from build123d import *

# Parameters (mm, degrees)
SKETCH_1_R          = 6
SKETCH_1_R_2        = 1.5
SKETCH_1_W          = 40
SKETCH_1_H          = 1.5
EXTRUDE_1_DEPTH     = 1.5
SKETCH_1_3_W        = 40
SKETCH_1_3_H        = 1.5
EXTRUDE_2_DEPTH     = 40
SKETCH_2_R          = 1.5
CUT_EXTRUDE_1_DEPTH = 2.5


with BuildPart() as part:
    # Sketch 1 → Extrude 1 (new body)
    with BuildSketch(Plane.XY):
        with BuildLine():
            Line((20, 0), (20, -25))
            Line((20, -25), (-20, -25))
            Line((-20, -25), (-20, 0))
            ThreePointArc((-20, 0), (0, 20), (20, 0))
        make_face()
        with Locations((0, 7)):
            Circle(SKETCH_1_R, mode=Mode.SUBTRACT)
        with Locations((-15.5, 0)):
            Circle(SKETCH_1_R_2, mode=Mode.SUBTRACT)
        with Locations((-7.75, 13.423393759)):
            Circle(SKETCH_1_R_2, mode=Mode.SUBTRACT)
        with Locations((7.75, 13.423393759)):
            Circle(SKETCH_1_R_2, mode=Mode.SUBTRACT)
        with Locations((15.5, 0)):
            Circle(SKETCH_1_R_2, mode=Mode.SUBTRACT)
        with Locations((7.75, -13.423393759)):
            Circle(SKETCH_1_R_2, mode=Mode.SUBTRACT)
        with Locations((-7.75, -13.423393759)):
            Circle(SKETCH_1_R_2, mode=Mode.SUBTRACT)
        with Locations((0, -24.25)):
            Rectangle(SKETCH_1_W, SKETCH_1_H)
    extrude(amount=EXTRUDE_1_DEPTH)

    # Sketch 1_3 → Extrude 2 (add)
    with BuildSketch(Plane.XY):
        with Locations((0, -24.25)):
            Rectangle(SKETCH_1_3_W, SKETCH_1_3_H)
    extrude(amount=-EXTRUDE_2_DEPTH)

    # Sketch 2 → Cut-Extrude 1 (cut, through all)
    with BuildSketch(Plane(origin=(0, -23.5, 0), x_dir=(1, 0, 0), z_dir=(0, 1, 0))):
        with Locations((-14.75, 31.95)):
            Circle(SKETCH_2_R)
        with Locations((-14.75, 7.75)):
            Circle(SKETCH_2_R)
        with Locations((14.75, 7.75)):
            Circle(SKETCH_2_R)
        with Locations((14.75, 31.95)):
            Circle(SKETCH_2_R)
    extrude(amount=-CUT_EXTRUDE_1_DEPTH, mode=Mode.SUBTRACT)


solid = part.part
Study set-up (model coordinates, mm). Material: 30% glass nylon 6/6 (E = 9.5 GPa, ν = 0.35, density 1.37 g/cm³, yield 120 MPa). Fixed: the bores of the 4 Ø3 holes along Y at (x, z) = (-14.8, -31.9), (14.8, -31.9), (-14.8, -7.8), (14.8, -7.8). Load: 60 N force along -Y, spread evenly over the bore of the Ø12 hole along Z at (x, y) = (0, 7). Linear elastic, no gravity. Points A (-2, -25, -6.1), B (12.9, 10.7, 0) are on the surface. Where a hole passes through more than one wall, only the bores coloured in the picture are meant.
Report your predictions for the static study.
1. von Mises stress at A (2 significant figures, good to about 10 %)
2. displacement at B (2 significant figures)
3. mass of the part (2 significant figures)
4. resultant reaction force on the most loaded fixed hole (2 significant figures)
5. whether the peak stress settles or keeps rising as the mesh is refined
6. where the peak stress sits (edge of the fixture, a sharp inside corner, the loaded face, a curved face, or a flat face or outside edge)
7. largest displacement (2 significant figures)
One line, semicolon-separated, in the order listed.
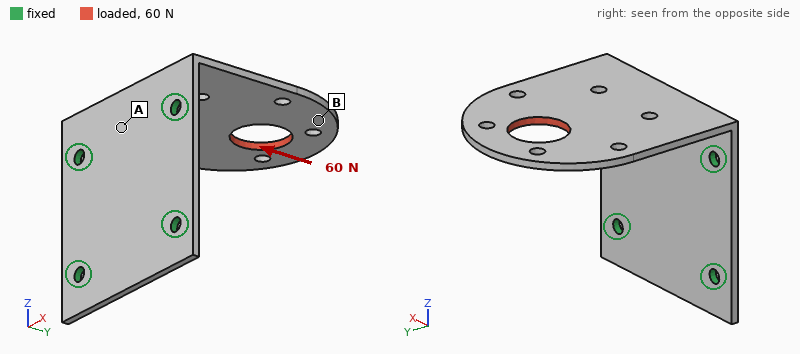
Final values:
8.6 MPa; 0.69 mm; 6.3 g; 32 N; keeps rising; edge of the fixture; 0.86 mm
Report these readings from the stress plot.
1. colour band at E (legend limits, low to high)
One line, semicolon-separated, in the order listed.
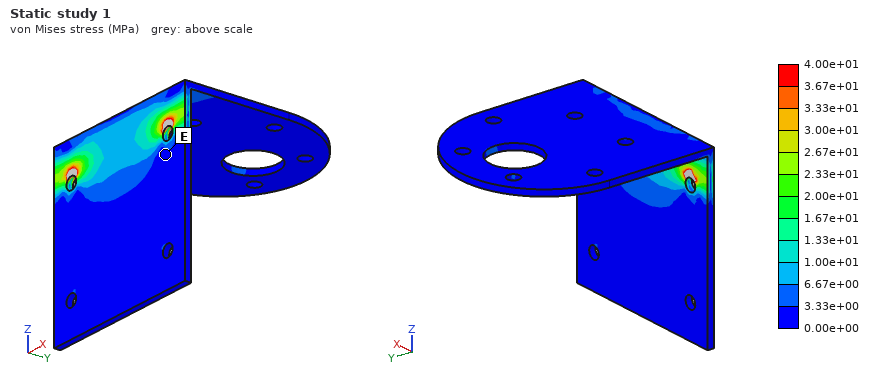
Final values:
0.00e+00 to 3.33e+00 MPa
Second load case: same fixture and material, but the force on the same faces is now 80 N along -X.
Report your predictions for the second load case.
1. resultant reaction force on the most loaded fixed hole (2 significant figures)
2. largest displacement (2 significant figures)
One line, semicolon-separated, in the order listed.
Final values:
95 N; 0.80 mm
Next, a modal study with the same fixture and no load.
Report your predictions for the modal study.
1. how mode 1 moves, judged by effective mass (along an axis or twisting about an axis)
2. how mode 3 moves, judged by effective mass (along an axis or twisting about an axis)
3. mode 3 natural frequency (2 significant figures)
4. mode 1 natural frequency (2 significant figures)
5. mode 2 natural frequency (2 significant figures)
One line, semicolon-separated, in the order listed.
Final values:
along Z; along X; 1500 Hz; 330 Hz; 940 Hz
